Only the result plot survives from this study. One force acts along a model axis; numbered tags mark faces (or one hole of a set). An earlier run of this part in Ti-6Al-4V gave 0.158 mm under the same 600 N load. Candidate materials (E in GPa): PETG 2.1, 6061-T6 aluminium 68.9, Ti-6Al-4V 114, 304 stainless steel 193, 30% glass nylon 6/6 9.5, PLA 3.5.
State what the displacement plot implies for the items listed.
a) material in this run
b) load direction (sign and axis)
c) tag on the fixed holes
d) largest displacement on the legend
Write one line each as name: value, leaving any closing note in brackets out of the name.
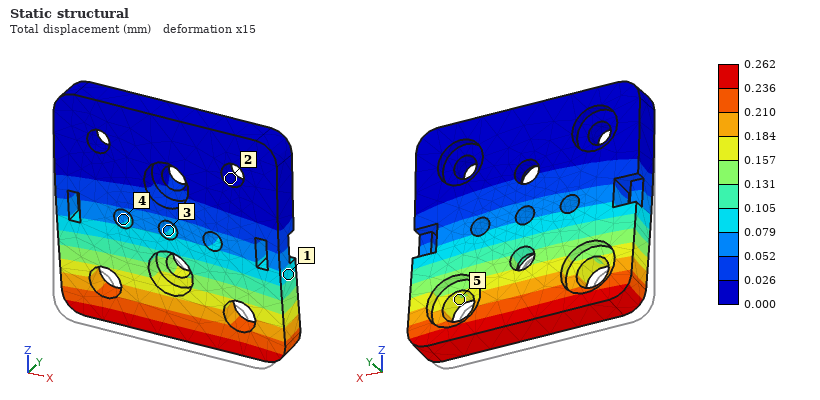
material in this run: 6061-T6 aluminium
load direction: +Y
tag on the fixed holes: 2
largest displacement on the legend: 0.262 mm
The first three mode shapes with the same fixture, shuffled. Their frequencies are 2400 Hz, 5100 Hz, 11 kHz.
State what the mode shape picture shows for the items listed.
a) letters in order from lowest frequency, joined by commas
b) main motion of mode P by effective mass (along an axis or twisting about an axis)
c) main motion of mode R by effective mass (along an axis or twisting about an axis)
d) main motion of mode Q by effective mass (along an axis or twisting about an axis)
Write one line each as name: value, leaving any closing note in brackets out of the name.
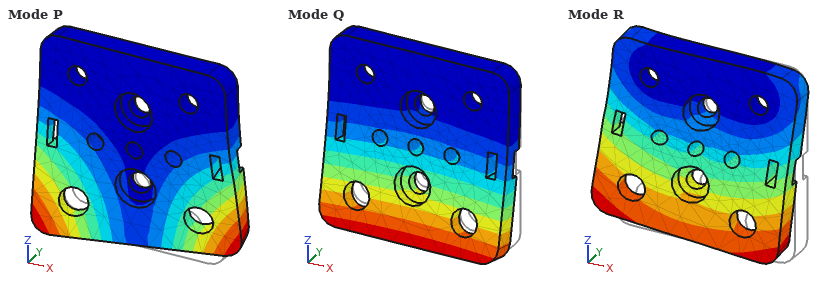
letters in order from lowest frequency, joined by commas: Q, P, R
main motion of mode P by effective mass: twisting about Z
main motion of mode R by effective mass: along X
main motion of mode Q by effective mass: along Y
